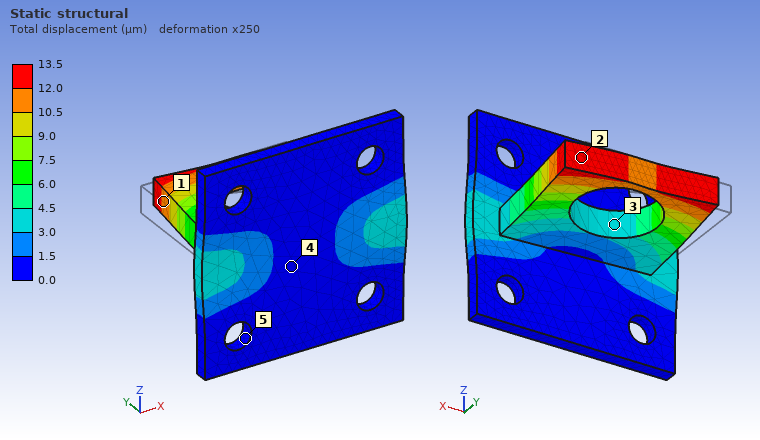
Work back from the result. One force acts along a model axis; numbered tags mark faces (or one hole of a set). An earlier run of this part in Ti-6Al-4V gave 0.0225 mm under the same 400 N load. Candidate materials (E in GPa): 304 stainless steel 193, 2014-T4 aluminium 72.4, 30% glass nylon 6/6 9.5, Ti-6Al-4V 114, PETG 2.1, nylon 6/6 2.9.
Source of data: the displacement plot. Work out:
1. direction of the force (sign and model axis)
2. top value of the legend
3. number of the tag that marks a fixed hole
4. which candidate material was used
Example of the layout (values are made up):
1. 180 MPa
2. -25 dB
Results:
1. +X
2. 13.5 µm
3. 5
4. 304 stainless steel
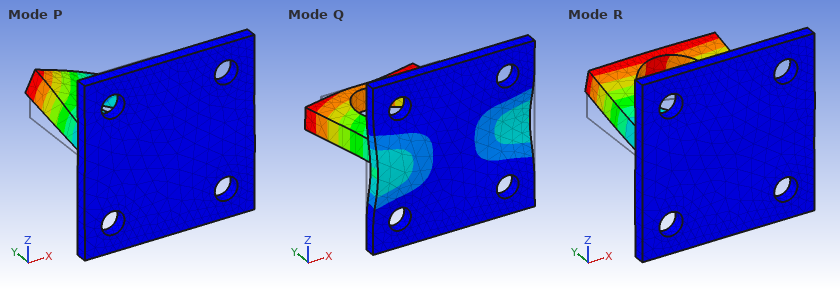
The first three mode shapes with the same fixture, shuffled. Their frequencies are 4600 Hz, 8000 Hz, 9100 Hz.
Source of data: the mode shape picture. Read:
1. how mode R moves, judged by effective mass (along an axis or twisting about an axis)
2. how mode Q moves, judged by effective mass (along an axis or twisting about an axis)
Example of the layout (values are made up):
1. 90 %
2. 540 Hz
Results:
1. along Z
2. along X
